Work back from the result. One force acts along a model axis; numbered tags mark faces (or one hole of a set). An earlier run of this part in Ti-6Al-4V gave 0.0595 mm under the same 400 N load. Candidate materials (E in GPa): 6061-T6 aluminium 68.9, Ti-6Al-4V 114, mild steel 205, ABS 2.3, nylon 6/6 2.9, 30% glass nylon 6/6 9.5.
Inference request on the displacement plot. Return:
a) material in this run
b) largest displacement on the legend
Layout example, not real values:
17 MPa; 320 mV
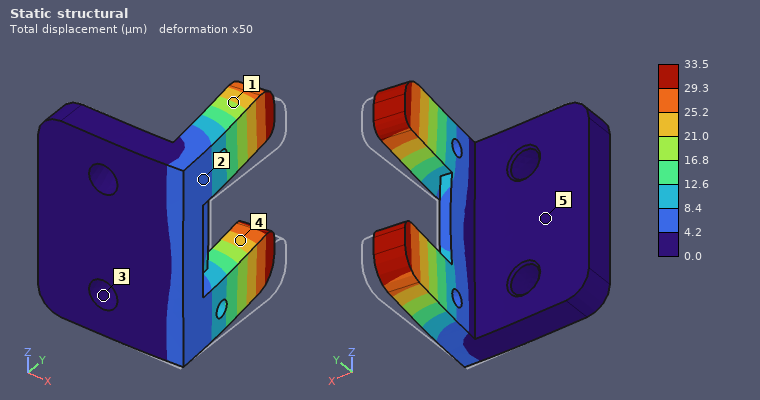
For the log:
mild steel; 33.5 µm
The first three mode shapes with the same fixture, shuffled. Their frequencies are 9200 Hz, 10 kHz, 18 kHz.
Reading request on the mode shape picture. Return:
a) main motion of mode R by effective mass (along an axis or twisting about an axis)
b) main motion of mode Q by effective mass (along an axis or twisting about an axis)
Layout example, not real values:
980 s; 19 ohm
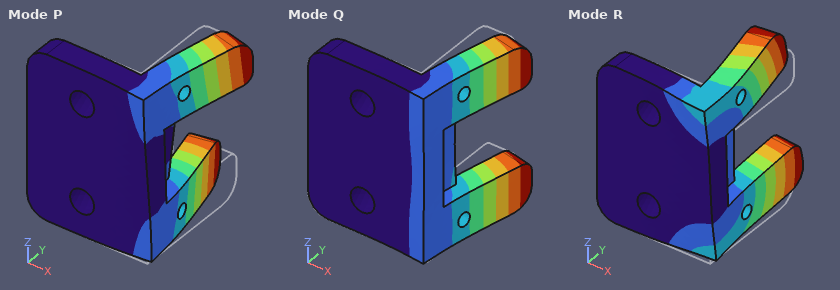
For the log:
along Z; along X
